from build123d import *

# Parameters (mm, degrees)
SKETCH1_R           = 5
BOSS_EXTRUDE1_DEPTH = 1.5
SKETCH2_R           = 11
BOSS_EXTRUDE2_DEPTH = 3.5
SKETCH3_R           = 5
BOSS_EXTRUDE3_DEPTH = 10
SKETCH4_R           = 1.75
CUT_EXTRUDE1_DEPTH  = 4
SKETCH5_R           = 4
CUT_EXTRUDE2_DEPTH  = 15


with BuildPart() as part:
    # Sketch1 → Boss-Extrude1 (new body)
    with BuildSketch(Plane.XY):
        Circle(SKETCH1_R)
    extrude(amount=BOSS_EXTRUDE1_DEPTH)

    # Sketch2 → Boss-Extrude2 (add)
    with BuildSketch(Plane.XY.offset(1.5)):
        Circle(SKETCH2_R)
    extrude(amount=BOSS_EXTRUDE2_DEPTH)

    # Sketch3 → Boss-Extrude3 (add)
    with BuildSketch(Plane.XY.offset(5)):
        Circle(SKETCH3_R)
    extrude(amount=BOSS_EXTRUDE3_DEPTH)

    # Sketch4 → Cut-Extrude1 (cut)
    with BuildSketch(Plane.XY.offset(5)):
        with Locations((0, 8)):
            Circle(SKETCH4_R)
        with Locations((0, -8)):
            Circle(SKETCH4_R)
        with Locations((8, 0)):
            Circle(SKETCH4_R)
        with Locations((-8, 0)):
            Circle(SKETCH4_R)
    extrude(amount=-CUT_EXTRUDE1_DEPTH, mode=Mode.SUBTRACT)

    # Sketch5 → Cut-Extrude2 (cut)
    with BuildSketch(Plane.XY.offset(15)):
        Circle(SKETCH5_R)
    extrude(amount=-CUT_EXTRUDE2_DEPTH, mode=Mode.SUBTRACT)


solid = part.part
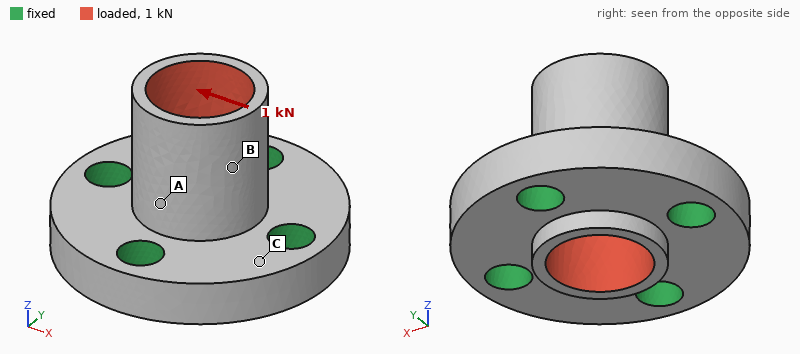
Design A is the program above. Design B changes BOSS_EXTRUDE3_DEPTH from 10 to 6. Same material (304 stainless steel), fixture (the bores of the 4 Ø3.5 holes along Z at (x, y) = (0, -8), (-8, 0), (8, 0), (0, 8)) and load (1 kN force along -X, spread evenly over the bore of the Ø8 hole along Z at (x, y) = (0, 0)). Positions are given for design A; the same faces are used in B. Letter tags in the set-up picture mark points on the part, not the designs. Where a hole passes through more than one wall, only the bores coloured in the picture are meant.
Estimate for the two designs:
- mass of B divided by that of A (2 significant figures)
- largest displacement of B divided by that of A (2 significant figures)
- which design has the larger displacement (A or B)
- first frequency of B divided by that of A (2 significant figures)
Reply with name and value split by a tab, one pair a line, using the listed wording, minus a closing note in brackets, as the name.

mass of B divided by that of A	0.92
largest displacement of B divided by that of A	0.44
which design has the larger displacement	A
first frequency of B divided by that of A	1.4
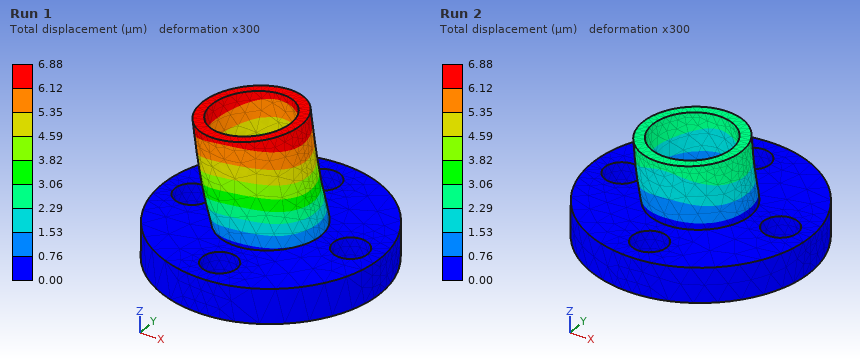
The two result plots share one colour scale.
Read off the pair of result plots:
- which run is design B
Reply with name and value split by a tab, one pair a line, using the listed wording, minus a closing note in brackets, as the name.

which run is design B	Run 2
